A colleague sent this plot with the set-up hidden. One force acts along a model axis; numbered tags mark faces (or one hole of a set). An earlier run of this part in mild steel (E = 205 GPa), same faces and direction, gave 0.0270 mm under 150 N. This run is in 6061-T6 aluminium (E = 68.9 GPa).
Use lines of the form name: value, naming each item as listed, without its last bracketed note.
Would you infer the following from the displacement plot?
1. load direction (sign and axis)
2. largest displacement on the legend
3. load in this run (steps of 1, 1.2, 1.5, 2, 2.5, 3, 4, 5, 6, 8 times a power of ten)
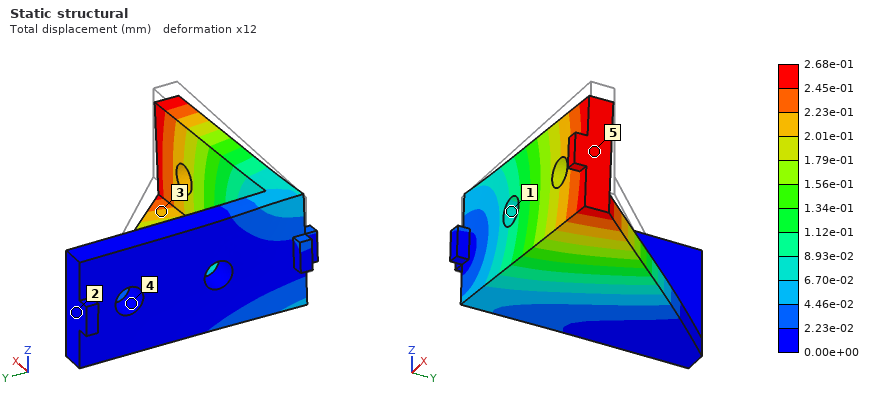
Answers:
load direction: -Z
largest displacement on the legend: 2.68e-01 mm
load in this run: 500 N
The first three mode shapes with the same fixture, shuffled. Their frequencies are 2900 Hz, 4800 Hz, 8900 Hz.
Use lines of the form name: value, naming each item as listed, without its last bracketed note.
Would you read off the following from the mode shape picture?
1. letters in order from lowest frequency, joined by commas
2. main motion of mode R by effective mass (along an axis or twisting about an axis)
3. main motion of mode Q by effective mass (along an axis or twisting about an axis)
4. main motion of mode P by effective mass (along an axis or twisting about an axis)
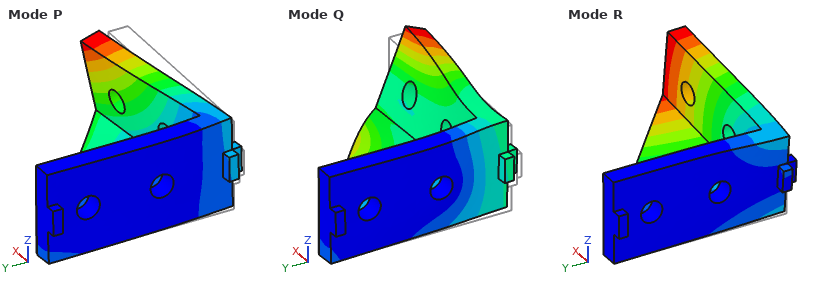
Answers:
letters in order from lowest frequency, joined by commas: R, P, Q
main motion of mode R by effective mass: along Z
main motion of mode Q by effective mass: along X
main motion of mode P by effective mass: along Y
